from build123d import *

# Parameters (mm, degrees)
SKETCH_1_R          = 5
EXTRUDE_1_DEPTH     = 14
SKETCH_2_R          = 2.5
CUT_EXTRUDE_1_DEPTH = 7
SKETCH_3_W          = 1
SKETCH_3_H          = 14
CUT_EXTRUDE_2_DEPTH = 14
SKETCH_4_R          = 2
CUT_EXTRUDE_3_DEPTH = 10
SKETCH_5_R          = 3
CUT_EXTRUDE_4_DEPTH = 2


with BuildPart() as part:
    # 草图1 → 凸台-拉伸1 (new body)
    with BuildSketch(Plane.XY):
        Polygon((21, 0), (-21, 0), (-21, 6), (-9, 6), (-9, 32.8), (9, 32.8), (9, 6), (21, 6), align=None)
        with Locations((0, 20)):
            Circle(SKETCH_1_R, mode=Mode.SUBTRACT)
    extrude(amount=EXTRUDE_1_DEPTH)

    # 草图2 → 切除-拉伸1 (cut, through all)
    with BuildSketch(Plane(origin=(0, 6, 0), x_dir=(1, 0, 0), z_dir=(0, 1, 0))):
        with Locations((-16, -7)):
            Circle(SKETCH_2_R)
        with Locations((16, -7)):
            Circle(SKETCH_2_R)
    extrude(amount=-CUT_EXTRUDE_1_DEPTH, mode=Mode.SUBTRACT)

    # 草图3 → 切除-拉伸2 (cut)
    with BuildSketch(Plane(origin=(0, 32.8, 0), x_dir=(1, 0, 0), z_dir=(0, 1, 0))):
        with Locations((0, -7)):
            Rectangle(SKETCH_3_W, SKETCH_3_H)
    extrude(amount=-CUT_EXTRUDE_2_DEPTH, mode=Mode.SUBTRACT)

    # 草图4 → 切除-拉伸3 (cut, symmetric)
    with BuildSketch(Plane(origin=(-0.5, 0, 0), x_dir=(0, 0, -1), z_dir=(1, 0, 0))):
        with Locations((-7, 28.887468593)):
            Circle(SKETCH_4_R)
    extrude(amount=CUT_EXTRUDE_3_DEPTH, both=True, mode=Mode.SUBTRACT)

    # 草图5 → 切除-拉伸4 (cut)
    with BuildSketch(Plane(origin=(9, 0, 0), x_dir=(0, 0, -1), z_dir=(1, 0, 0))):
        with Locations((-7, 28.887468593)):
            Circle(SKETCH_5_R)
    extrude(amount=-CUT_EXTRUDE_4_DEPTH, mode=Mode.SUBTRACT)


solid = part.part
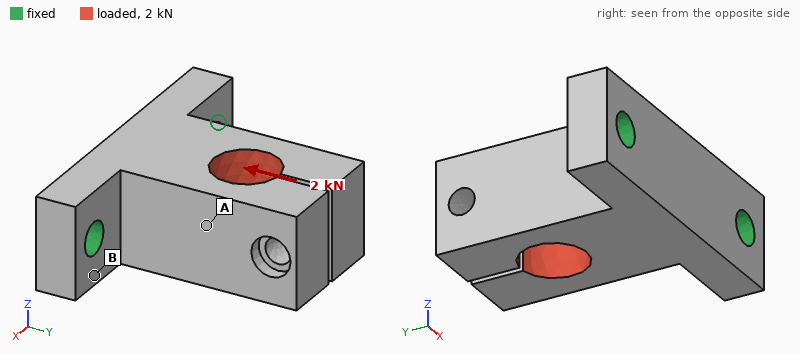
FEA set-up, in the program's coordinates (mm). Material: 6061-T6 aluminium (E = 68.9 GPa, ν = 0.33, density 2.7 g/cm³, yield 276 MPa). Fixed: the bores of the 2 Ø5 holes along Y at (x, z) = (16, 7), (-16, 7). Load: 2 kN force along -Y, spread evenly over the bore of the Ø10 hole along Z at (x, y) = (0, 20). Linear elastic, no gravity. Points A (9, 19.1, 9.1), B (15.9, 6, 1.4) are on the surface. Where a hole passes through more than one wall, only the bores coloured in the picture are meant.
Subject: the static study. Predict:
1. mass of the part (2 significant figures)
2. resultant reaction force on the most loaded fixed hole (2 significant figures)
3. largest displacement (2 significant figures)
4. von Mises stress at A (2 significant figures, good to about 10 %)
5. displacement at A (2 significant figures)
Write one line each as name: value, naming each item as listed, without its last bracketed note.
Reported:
mass of the part: 23 g
resultant reaction force on the most loaded fixed hole: 1.1 kN
largest displacement: 43 µm
von Mises stress at A: 30 MPa
displacement at A: 6.8 µm
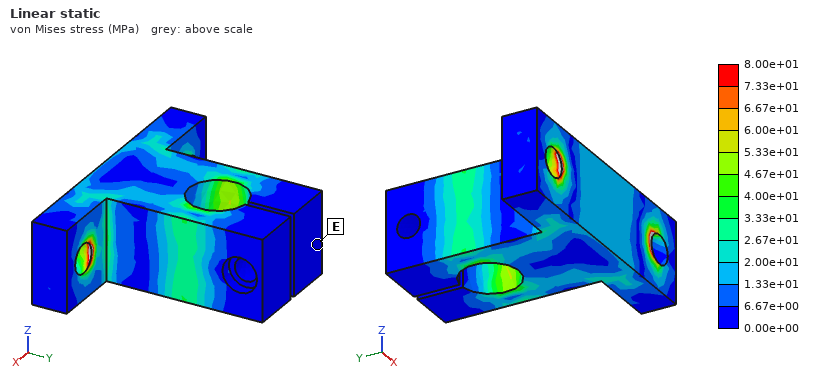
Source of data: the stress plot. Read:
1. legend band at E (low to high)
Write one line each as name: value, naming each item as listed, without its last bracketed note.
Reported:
legend band at E: 0.00e+00 to 6.67e+00 MPa
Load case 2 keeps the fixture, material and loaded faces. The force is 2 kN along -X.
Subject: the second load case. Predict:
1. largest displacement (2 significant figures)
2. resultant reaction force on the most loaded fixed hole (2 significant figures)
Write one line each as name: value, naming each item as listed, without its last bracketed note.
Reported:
largest displacement: 85 µm
resultant reaction force on the most loaded fixed hole: 1.7 kN
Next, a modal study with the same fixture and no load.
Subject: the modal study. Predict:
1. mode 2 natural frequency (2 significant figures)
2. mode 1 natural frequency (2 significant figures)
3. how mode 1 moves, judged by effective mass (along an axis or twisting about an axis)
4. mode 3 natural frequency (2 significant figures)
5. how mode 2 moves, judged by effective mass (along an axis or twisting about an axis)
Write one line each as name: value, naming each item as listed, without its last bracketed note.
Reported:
mode 2 natural frequency: 6900 Hz
mode 1 natural frequency: 5100 Hz
how mode 1 moves, judged by effective mass: along Z
mode 3 natural frequency: 7700 Hz
how mode 2 moves, judged by effective mass: along X
